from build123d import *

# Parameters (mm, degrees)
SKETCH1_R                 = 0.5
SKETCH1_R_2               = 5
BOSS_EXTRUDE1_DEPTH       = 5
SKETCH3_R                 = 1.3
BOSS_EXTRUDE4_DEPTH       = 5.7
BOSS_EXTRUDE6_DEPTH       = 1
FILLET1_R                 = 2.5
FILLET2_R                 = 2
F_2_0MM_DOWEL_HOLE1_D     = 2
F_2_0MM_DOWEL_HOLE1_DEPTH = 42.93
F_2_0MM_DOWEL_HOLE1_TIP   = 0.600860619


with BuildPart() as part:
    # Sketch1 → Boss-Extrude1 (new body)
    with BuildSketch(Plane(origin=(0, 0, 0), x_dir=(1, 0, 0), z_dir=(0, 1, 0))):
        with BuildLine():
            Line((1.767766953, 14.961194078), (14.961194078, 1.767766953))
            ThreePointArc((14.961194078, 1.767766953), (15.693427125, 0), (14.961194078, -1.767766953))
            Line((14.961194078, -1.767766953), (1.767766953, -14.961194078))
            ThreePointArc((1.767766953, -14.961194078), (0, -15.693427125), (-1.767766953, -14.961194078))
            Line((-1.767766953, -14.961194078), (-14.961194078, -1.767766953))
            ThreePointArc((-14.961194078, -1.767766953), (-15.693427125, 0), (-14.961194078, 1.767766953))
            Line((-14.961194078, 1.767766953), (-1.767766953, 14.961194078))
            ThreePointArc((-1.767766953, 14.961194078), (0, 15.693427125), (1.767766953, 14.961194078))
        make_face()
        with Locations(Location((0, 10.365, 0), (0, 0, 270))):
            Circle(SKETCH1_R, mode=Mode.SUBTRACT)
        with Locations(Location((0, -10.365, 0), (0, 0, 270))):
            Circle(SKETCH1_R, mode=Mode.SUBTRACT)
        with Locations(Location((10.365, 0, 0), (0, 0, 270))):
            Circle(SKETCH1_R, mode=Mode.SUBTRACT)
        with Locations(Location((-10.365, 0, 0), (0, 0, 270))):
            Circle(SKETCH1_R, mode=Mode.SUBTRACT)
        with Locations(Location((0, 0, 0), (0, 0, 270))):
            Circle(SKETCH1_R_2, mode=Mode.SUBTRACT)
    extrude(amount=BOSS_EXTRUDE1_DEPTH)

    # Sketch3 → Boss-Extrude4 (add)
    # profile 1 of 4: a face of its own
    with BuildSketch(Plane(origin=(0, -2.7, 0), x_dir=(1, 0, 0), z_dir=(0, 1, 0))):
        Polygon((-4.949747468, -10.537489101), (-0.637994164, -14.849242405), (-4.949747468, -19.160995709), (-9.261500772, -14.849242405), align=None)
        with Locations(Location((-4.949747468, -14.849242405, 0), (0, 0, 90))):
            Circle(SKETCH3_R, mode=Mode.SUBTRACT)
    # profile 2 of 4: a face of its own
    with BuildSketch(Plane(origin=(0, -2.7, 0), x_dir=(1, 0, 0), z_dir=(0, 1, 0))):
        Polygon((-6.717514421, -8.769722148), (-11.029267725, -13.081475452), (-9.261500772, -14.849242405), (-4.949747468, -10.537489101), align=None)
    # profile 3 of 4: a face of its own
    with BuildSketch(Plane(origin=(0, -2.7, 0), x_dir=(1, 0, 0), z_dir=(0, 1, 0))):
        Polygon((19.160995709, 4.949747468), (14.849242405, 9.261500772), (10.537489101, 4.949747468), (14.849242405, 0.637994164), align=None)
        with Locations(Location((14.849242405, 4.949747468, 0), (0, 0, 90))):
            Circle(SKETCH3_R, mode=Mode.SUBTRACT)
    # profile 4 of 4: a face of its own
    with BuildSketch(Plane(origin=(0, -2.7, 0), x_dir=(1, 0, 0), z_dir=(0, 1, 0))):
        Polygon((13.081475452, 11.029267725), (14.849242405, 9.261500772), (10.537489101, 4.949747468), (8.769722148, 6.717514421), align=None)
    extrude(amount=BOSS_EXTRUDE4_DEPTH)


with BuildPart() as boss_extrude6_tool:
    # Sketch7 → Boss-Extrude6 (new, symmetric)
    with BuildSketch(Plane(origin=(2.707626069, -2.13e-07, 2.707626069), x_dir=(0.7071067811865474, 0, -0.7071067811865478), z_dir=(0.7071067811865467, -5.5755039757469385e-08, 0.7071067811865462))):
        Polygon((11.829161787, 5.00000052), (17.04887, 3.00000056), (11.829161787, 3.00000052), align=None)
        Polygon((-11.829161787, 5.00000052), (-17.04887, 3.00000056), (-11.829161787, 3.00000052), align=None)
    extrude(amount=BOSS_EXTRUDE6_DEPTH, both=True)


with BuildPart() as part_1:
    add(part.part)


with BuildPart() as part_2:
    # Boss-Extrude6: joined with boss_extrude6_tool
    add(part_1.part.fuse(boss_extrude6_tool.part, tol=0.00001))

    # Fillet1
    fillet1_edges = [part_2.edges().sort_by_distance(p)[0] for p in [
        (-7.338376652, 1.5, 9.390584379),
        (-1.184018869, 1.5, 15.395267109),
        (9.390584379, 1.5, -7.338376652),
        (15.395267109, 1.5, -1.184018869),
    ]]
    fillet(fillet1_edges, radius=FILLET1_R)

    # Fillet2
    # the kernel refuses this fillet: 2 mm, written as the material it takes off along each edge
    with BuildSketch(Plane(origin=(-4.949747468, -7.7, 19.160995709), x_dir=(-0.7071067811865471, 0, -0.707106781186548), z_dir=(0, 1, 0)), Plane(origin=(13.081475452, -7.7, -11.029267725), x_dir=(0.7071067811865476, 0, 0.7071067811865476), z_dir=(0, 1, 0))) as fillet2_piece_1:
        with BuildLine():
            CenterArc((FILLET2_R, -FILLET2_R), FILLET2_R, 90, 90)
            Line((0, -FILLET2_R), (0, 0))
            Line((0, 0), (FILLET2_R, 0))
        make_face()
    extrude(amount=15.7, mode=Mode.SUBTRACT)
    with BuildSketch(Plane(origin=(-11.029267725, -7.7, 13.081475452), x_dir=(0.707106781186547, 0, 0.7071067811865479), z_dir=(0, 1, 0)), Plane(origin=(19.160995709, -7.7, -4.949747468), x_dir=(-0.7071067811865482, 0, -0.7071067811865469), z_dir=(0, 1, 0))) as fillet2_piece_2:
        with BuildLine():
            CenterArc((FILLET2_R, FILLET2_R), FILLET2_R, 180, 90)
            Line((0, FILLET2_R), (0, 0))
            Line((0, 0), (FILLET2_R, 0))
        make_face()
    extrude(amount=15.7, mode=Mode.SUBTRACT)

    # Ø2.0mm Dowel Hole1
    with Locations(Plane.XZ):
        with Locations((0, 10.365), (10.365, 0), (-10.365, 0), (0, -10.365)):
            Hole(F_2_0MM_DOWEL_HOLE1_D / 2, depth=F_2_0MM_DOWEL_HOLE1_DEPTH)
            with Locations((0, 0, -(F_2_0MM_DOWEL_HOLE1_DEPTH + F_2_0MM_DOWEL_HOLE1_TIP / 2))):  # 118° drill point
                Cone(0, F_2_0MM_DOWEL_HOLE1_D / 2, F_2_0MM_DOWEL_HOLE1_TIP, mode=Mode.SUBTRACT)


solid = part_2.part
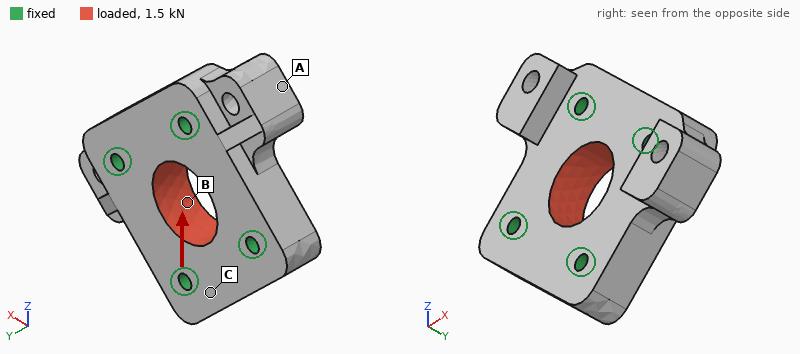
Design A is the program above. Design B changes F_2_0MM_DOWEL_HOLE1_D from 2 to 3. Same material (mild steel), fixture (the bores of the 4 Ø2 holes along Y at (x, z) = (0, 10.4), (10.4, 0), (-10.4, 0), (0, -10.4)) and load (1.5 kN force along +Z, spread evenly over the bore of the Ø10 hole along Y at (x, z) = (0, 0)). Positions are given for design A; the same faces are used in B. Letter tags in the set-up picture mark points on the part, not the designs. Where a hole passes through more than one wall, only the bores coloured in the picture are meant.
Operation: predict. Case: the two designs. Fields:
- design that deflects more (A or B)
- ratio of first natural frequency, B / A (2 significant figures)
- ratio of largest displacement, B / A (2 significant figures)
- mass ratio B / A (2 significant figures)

A
1.1
0.86
0.97
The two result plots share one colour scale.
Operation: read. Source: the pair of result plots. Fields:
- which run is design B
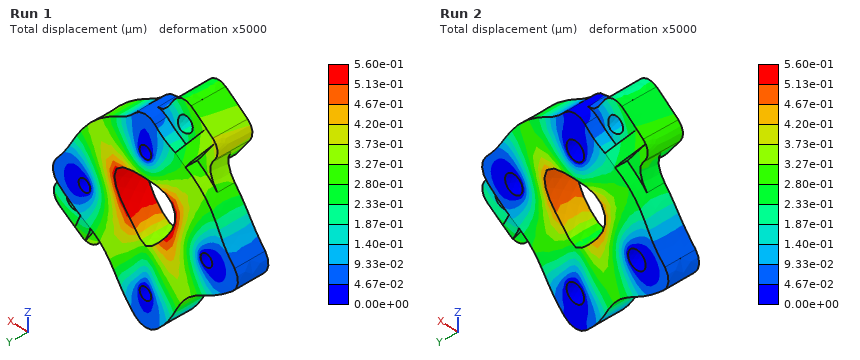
Run 2
